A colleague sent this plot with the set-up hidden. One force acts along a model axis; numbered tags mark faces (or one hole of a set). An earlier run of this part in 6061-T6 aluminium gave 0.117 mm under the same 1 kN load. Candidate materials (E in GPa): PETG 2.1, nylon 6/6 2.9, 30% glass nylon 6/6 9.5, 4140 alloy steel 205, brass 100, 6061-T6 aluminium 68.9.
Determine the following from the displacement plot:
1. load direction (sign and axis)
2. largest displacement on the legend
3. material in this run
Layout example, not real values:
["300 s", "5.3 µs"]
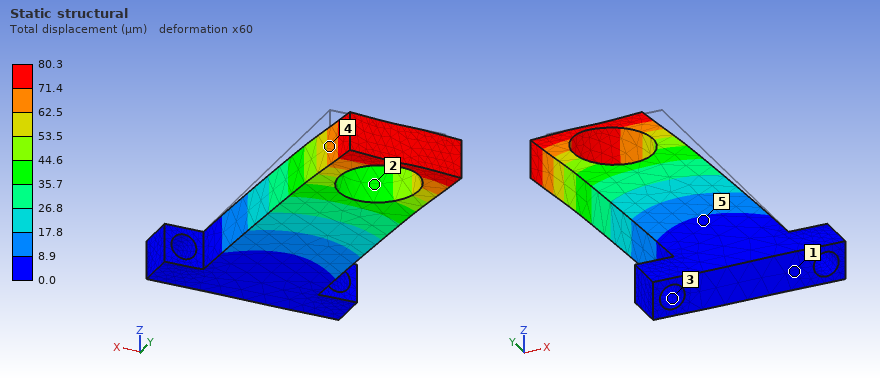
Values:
["-X", "80.3 µm", "brass"]
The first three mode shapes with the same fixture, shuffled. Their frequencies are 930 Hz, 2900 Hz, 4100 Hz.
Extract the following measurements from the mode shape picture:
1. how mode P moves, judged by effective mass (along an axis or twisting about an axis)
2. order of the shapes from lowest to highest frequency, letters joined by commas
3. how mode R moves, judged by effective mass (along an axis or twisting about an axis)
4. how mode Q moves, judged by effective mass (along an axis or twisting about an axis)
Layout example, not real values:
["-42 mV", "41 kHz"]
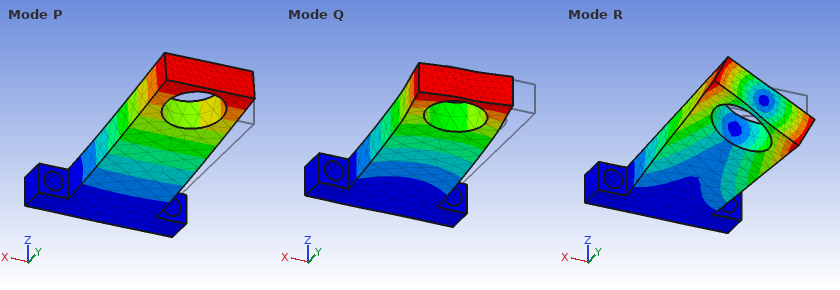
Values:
["along Z", "P, Q, R", "twisting about Y", "along X"]
